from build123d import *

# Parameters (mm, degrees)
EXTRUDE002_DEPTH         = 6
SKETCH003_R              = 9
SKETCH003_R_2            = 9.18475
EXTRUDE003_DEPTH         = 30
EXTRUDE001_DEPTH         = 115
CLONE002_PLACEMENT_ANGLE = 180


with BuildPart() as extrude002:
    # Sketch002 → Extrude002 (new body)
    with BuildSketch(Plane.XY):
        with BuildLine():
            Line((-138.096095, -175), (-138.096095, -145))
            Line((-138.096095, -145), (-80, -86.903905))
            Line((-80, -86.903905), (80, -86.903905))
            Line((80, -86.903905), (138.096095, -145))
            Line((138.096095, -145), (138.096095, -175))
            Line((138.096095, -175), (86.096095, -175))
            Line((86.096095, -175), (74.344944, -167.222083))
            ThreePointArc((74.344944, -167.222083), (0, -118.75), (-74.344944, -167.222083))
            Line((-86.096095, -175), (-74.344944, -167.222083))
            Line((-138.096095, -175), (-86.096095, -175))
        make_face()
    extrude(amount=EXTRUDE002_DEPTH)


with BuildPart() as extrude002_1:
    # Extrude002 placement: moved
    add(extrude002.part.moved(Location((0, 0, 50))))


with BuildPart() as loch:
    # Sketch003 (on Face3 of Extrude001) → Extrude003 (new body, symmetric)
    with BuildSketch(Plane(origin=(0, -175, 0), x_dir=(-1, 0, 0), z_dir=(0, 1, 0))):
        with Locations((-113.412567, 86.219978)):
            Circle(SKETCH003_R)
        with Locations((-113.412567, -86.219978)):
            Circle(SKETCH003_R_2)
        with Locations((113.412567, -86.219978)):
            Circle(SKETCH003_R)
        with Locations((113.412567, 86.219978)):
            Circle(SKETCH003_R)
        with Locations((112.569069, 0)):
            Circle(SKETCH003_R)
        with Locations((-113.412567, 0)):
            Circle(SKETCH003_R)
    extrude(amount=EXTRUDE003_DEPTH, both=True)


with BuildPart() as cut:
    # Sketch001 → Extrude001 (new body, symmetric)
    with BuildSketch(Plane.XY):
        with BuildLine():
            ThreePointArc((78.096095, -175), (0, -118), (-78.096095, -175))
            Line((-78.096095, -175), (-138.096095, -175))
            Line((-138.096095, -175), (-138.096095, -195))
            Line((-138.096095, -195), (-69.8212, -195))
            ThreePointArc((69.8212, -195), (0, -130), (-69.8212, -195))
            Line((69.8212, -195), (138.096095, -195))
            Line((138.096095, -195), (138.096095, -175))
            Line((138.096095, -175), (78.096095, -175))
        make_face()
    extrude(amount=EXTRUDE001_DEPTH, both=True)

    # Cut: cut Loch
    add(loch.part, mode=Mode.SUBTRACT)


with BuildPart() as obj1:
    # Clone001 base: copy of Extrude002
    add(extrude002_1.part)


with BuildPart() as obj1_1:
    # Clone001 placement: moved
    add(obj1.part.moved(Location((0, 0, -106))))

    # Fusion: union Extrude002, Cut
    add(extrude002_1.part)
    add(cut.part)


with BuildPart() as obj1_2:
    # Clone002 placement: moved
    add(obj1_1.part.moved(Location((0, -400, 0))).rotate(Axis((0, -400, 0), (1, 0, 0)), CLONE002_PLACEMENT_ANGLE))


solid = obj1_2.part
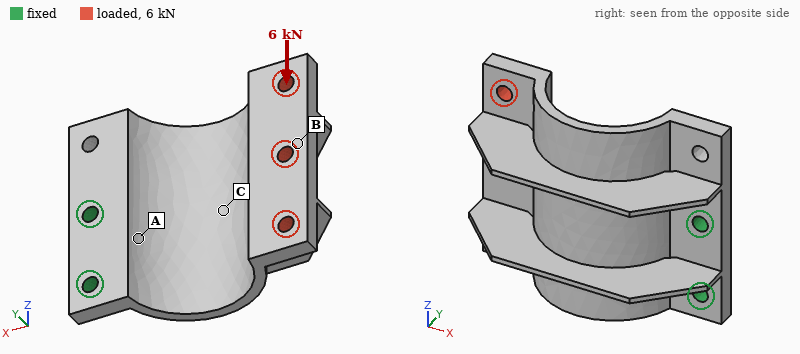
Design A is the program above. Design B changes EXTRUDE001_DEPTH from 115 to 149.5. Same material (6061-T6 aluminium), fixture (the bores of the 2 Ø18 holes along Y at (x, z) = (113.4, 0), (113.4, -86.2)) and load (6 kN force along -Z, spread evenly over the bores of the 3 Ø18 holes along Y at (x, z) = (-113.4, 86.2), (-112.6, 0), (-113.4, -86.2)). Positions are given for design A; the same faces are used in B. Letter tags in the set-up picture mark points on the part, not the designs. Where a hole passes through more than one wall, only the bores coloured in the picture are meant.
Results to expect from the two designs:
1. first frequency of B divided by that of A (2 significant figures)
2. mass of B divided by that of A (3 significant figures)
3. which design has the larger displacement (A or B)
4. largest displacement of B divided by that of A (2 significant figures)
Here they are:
0.89
1.27
A
0.91
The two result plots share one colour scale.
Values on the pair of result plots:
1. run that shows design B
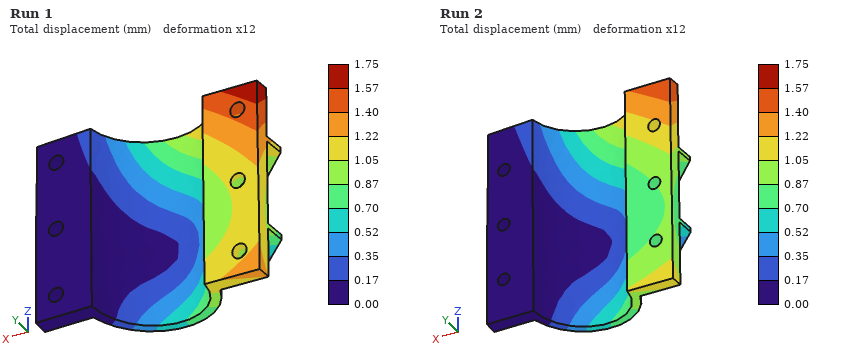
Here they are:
Run 2
